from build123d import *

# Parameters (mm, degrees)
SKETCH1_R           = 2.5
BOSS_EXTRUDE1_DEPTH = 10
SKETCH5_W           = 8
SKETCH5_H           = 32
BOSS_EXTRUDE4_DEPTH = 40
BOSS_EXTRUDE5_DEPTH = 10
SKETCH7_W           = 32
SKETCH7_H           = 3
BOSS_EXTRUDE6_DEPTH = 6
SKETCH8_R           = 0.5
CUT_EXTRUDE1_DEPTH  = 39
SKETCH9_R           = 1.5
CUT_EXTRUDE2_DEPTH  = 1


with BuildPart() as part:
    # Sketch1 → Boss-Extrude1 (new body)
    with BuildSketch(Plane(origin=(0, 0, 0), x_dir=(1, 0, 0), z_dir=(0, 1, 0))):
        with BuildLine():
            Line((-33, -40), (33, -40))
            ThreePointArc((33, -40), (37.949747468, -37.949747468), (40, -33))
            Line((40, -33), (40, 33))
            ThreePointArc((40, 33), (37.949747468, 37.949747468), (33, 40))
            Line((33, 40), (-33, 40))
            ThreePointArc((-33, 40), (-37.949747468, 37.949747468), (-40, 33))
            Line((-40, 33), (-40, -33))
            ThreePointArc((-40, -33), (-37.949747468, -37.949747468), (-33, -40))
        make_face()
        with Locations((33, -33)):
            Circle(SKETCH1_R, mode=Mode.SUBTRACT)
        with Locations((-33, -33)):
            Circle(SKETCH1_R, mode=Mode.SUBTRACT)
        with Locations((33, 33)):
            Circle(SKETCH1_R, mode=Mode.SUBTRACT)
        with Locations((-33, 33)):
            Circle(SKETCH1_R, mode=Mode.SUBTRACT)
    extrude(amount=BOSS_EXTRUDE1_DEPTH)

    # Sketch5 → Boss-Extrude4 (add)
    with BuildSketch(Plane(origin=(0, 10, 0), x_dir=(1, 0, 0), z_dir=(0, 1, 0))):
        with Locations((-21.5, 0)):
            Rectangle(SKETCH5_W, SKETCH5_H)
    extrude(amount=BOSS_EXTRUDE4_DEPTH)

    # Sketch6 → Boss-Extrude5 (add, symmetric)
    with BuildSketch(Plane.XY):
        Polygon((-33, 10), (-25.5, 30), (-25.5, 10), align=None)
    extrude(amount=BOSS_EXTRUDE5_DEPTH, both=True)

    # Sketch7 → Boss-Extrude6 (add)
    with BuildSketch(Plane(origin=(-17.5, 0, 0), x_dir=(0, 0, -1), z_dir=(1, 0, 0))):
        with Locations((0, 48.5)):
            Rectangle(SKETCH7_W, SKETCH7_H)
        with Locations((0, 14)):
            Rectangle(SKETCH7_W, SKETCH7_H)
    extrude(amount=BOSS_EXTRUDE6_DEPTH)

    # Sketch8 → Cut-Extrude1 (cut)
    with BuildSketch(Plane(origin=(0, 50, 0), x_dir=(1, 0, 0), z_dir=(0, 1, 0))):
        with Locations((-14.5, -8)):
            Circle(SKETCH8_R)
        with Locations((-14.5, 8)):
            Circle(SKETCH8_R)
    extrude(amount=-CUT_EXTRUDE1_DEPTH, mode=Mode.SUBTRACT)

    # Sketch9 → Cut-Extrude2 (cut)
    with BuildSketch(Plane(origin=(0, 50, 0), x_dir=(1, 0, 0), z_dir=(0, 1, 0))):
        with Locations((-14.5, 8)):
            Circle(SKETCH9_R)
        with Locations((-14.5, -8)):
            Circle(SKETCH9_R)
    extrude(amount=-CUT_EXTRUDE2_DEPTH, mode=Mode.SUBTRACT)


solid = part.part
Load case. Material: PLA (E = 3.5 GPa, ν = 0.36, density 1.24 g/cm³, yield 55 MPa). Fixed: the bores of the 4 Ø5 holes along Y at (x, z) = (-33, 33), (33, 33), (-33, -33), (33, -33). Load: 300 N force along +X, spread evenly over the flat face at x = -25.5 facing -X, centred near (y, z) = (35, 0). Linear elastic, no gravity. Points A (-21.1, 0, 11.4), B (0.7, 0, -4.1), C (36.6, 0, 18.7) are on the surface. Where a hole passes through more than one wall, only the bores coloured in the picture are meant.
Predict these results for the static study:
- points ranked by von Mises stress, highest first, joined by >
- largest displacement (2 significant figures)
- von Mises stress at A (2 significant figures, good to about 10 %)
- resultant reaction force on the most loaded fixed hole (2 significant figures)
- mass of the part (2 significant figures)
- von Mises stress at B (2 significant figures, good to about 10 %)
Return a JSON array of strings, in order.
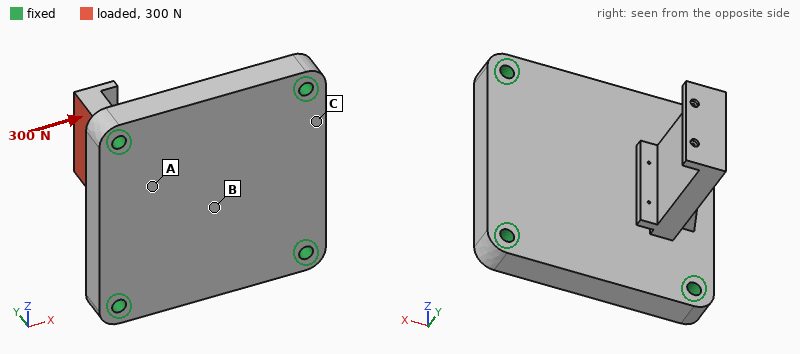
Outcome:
["A > B > C", "0.57 mm", "3.4 MPa", "110 N", "94 g", "1.8 MPa"]
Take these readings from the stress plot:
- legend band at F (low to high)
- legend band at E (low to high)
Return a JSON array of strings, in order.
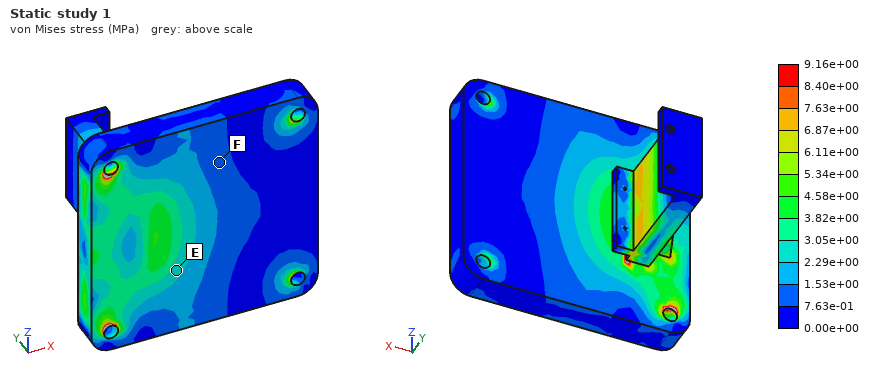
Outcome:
["7.63e-01 to 1.53e+00 MPa", "2.29e+00 to 3.05e+00 MPa"]
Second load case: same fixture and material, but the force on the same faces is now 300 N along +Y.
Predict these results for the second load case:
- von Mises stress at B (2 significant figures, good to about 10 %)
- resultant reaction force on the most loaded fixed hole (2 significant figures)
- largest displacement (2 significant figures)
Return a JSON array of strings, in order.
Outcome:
["0.66 MPa", "140 N", "0.11 mm"]
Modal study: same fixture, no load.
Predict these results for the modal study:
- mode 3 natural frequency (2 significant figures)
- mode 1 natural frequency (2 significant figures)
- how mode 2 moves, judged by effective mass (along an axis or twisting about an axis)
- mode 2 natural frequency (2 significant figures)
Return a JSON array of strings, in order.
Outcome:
["2400 Hz", "1300 Hz", "along Y", "2200 Hz"]
